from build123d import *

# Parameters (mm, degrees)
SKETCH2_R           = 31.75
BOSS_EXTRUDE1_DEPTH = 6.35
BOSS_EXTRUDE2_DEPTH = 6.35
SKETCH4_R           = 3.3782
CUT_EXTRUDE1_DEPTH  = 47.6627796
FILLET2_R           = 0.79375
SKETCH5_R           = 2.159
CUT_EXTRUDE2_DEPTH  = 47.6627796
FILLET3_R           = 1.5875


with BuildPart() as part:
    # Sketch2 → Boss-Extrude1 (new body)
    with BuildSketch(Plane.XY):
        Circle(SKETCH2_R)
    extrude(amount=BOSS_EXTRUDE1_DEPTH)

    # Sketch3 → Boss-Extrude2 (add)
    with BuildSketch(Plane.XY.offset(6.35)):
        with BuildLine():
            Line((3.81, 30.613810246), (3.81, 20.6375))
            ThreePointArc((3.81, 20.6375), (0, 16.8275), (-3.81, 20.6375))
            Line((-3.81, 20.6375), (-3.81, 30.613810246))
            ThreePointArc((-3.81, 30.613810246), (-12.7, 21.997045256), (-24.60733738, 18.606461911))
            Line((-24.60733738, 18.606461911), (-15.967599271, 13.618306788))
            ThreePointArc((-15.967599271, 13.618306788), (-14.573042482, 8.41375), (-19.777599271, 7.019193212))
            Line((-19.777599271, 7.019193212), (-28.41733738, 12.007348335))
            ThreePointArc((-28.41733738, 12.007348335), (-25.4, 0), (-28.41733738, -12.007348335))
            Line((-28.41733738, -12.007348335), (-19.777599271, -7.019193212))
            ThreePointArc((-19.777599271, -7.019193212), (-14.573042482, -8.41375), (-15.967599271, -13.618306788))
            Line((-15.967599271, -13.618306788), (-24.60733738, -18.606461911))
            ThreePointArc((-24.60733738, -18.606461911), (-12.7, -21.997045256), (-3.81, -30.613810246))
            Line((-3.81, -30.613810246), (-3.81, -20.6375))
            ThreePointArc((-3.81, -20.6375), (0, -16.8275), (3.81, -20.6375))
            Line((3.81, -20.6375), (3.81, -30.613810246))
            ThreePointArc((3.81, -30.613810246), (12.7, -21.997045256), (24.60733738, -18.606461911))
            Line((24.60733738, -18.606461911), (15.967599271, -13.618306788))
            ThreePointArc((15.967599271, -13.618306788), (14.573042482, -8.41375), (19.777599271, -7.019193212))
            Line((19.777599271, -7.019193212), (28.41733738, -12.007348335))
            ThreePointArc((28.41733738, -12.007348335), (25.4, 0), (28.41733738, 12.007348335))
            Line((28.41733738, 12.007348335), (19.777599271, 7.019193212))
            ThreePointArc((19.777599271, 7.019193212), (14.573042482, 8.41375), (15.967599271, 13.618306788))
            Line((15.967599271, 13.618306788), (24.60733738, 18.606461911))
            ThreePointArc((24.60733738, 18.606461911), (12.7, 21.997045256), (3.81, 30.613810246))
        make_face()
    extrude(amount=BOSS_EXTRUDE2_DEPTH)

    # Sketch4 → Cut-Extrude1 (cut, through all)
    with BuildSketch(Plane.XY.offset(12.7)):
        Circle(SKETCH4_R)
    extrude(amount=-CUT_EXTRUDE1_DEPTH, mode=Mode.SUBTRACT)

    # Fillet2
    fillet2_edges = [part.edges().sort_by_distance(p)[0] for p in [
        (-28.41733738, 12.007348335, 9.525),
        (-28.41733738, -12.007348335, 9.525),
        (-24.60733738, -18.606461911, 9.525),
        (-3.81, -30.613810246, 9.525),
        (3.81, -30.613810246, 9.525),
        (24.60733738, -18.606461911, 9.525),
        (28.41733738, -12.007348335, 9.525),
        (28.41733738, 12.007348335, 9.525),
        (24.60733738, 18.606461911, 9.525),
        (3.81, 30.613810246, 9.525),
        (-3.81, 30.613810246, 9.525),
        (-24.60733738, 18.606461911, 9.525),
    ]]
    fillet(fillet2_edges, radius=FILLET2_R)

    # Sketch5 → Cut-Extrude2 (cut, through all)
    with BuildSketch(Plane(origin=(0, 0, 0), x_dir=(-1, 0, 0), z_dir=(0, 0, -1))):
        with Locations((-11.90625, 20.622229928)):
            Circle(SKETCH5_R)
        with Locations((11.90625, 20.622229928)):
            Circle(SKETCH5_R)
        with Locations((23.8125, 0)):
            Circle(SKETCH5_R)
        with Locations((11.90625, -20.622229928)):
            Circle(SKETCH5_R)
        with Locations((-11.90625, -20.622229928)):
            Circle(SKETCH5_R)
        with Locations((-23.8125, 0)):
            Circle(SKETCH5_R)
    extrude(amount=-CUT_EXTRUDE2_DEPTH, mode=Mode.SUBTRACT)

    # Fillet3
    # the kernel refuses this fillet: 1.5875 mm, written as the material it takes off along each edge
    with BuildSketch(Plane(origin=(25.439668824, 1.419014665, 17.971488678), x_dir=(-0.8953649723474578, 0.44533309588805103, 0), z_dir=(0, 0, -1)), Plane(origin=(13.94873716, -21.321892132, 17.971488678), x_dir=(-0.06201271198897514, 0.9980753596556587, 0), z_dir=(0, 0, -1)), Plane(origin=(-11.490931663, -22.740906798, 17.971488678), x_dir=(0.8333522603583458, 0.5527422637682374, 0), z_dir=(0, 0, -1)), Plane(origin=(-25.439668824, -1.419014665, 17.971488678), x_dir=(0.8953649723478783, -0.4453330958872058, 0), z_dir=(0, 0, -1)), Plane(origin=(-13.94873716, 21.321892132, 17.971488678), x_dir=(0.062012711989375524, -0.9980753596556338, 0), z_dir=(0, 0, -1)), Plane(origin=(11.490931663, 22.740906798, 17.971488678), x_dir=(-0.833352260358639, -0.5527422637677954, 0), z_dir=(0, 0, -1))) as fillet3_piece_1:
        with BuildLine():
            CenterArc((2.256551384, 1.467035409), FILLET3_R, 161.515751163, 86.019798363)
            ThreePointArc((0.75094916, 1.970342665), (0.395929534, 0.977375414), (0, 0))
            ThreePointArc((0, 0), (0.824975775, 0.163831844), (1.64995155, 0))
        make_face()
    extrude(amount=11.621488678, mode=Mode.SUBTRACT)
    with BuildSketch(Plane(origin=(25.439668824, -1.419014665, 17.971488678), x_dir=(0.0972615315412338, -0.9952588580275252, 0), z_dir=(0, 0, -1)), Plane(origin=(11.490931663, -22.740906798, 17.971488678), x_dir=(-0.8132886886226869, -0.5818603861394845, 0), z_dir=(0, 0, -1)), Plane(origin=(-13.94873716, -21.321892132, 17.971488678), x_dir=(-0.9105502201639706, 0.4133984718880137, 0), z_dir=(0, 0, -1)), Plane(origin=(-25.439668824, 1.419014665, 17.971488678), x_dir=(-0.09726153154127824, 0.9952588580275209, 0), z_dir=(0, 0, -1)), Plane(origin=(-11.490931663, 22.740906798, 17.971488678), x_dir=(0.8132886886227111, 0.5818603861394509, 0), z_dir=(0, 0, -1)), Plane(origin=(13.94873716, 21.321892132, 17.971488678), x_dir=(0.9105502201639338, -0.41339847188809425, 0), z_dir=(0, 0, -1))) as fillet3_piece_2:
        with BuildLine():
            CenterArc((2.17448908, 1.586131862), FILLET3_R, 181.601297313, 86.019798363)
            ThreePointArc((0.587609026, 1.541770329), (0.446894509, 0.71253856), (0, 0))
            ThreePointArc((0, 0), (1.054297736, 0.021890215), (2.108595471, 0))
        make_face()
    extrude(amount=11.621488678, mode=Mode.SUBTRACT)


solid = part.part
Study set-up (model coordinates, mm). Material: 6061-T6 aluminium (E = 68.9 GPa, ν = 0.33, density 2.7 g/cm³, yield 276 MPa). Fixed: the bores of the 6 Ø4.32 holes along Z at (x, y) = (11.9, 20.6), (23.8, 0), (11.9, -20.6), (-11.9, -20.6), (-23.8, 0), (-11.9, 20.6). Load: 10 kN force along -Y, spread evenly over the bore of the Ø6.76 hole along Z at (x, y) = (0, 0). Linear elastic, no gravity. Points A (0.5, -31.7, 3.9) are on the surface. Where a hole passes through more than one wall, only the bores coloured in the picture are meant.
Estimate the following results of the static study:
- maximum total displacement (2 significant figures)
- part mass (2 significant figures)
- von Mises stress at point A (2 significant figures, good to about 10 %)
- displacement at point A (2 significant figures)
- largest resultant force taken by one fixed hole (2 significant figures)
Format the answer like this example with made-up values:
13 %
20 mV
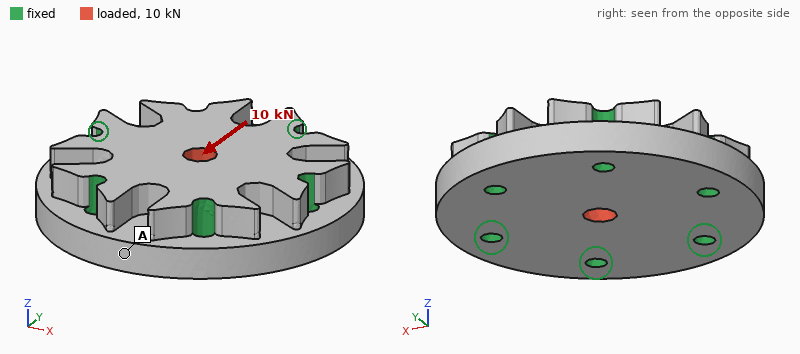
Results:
6.9 µm
82 g
7.4 MPa
1.5 µm
2.4 kN
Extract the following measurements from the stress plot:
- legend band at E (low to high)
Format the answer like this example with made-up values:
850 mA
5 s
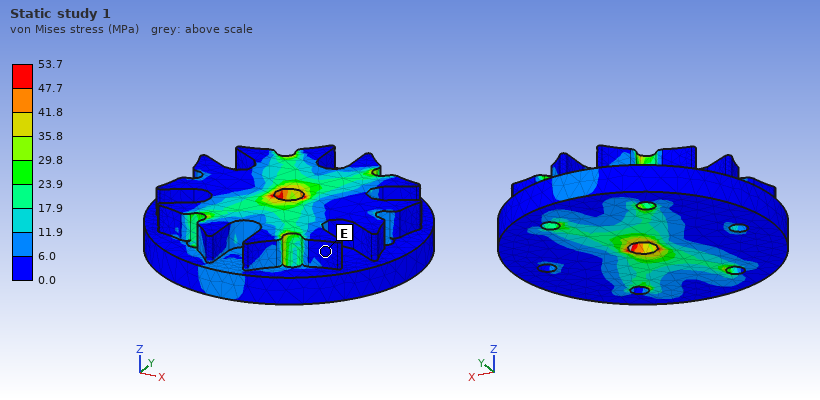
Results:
0.0 to 6.0 MPa
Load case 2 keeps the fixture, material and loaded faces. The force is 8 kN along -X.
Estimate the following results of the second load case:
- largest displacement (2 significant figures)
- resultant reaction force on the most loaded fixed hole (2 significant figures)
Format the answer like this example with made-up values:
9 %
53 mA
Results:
5.6 µm
2.2 kN
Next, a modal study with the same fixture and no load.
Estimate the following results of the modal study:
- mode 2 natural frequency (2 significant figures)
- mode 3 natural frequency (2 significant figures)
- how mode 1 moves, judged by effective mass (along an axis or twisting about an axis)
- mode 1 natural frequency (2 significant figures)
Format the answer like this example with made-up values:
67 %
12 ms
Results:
43 kHz
44 kHz
along Z
30 kHz
